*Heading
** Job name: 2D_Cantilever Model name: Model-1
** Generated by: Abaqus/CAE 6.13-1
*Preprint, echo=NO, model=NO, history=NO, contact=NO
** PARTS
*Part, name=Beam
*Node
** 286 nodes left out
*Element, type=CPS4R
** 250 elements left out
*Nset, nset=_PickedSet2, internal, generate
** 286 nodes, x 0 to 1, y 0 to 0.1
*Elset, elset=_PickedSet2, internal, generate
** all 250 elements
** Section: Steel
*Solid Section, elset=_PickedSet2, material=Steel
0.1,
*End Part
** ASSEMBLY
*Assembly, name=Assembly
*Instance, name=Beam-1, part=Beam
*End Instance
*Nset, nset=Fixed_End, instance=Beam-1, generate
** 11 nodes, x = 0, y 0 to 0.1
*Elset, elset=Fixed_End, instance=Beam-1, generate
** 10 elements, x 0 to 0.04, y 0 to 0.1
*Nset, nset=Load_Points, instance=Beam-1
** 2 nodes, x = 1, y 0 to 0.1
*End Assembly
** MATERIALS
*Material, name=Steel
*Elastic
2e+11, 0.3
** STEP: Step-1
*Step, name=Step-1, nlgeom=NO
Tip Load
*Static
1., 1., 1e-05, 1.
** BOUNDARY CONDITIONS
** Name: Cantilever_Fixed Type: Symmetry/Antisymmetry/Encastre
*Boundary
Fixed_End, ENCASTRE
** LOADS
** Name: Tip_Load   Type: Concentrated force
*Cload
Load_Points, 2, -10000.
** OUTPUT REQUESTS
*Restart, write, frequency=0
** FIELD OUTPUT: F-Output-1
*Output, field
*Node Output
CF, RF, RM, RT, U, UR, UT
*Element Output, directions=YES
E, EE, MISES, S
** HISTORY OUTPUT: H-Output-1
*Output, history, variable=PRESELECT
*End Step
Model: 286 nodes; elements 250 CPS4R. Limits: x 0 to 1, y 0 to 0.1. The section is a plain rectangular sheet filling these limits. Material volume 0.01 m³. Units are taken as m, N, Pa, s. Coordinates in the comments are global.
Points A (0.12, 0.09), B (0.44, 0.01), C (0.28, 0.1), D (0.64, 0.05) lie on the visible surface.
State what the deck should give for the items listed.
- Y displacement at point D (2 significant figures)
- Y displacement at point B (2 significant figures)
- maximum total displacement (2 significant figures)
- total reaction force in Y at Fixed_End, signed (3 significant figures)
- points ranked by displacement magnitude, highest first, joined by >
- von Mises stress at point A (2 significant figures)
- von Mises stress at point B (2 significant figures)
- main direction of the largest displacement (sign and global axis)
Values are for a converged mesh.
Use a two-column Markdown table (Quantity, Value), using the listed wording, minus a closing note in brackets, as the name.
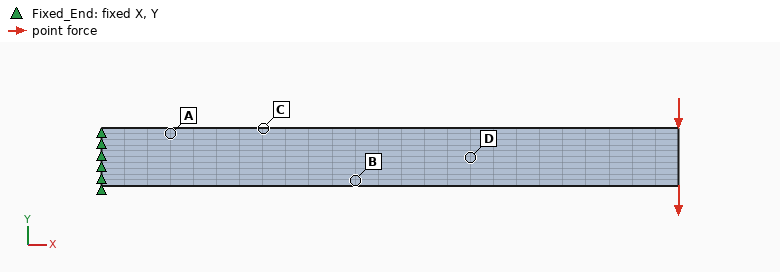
| Quantity | Value |
|---|---|
| Y displacement at point D | -0.0019 m |
| Y displacement at point B | -9.8e-04 m |
| maximum total displacement | 0.0039 m |
| total reaction force in Y at Fixed_End, signed | 20000 N |
| points ranked by displacement magnitude, highest first, joined by > | D > B > C > A |
| von Mises stress at point A | 8.2e+07 Pa |
| von Mises stress at point B | 5.2e+07 Pa |
| main direction of the largest displacement | -Y |
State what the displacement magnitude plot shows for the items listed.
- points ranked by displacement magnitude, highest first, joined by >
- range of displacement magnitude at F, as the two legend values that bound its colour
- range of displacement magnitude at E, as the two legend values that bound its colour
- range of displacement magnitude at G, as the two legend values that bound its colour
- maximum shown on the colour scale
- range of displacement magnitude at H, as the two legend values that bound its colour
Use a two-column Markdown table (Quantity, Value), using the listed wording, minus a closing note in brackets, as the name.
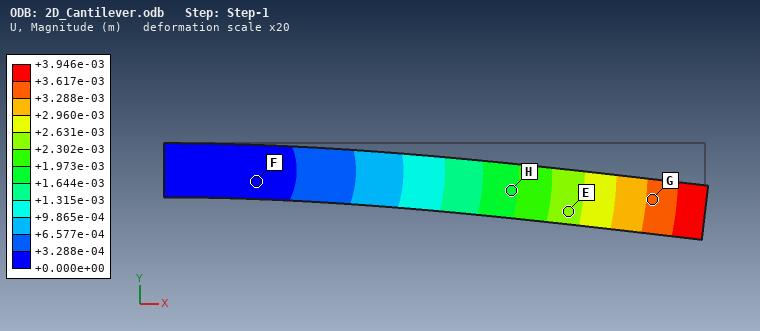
| Quantity | Value |
|---|---|
| points ranked by displacement magnitude, highest first, joined by > | G > E > H > F |
| range of displacement magnitude at F, as the two legend values that bound its colour | +0.000e+00 to +3.288e-04 m |
| range of displacement magnitude at E, as the two legend values that bound its colour | +2.302e-03 to +2.631e-03 m |
| range of displacement magnitude at G, as the two legend values that bound its colour | +3.288e-03 to +3.617e-03 m |
| maximum shown on the colour scale | +3.946e-03 m |
| range of displacement magnitude at H, as the two legend values that bound its colour | +1.644e-03 to +1.973e-03 m |
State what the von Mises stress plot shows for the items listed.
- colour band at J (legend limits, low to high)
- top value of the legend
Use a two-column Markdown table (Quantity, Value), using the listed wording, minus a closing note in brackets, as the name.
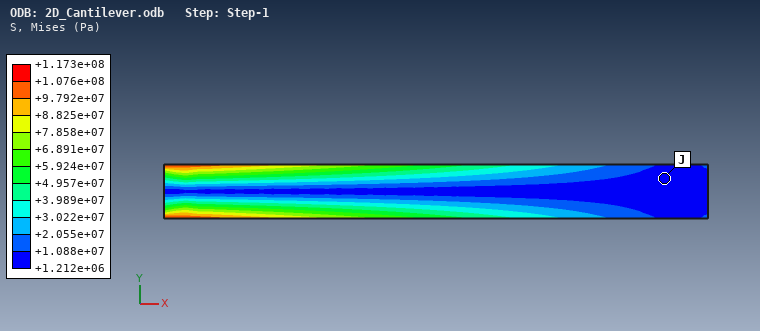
| Quantity | Value |
|---|---|
| colour band at J | +1.212e+06 to +1.088e+07 Pa |
| top value of the legend | +1.173e+08 Pa |
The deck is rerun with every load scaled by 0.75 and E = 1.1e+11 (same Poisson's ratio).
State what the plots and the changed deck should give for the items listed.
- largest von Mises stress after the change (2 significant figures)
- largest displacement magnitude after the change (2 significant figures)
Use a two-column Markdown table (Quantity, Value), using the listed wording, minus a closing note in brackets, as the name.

| Quantity | Value |
|---|---|
| largest von Mises stress after the change | 8.8e+07 Pa |
| largest displacement magnitude after the change | 0.0054 m |
